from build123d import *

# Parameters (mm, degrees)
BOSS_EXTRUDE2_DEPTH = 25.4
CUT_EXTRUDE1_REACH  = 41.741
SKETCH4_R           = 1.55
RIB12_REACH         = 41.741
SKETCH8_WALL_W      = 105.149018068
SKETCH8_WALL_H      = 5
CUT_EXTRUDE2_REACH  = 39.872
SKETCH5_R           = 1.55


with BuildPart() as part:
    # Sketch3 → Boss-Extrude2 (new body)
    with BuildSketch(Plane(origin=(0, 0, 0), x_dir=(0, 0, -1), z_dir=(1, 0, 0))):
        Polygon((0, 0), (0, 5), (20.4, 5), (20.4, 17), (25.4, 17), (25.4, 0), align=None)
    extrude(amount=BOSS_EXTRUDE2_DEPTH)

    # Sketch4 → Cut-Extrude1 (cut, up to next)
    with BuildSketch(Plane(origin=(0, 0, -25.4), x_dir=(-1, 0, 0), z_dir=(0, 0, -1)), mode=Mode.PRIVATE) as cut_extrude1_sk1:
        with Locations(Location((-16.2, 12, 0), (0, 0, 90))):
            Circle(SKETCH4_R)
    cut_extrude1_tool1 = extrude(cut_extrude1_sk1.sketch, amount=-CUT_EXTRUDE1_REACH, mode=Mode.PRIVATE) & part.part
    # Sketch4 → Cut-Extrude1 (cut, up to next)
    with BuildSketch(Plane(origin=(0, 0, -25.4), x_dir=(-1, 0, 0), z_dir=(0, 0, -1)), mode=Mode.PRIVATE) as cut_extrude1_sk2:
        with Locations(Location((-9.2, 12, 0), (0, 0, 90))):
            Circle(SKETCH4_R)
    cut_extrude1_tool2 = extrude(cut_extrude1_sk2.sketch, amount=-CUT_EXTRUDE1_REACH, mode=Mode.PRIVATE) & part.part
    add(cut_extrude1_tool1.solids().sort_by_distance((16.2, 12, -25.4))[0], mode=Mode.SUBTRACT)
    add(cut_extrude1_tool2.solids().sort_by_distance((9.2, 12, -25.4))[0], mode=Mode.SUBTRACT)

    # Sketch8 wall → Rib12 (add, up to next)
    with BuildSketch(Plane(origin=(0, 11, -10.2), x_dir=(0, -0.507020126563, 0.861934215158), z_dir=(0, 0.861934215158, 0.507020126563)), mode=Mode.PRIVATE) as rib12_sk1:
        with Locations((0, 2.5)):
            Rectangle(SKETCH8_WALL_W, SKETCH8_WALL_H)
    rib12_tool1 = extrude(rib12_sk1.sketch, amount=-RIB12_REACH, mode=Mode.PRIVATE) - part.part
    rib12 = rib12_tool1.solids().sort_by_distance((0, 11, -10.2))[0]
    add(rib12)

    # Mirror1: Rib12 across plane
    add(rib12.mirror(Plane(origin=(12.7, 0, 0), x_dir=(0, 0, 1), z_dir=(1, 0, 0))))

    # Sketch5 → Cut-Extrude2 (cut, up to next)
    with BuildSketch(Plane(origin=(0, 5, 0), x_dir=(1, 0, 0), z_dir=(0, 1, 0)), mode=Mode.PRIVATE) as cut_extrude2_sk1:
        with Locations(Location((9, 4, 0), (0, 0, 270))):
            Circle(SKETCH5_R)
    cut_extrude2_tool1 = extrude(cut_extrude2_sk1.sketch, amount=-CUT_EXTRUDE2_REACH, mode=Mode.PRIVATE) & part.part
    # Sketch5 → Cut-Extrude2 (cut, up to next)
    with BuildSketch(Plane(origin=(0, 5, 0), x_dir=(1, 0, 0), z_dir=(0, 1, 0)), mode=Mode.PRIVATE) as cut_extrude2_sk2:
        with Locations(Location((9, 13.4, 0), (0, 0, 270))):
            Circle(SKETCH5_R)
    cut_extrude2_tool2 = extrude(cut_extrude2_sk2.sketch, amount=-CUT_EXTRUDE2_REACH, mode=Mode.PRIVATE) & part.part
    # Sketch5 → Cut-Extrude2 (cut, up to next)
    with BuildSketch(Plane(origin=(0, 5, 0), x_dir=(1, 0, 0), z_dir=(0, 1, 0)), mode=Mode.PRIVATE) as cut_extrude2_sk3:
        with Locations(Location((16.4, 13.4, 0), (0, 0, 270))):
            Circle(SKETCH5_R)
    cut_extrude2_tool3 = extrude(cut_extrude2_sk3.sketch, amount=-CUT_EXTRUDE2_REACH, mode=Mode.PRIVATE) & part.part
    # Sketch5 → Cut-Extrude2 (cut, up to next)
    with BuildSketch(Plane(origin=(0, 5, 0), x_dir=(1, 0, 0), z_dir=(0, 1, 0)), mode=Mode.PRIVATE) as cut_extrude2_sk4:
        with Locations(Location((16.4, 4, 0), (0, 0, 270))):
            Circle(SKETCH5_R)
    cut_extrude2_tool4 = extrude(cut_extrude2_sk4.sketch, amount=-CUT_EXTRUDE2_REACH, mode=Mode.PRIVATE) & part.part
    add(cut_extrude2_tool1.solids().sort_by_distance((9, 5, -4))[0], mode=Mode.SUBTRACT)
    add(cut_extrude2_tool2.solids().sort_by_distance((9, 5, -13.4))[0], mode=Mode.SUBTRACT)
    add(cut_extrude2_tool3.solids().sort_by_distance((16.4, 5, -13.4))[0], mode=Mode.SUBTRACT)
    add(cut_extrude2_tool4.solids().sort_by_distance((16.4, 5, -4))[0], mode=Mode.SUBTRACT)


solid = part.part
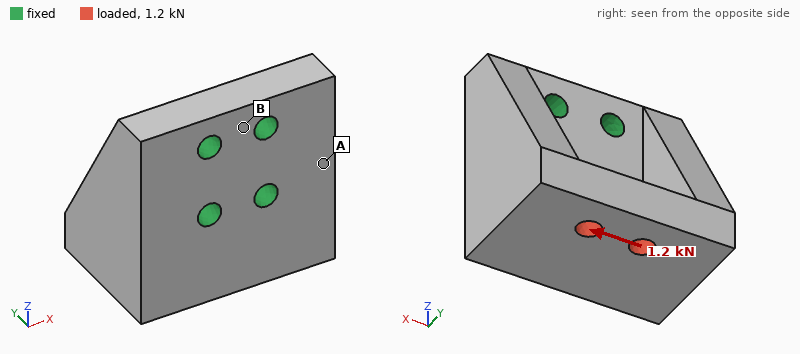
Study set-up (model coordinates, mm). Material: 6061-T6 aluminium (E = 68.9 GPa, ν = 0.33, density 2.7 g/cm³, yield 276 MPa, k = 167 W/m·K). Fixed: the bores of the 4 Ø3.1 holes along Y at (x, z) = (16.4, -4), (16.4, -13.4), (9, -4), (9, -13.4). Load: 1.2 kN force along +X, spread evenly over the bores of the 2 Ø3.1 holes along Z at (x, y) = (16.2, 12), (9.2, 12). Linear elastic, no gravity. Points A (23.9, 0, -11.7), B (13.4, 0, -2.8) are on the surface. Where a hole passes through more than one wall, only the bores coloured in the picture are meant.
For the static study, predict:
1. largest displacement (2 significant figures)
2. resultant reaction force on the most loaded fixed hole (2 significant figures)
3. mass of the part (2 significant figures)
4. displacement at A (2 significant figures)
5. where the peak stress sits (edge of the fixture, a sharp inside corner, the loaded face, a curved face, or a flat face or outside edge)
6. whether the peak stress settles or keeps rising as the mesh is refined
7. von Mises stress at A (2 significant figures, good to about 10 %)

35 µm
1.1 kN
16 g
8.0 µm
edge of the fixture
keeps rising
22 MPa
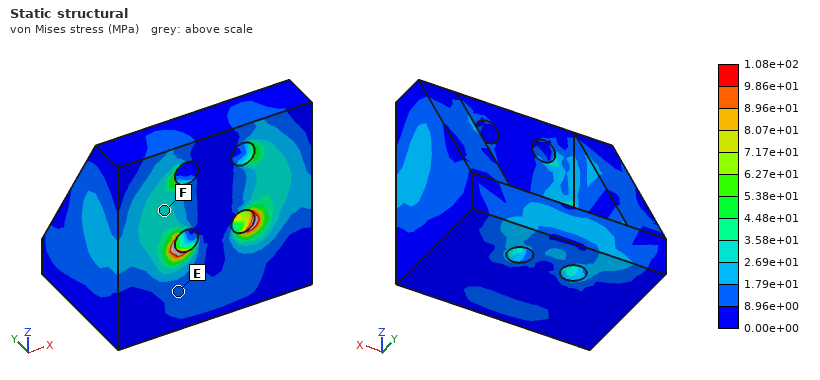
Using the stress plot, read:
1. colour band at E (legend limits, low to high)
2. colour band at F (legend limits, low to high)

8.96e+00 to 1.79e+01 MPa
2.69e+01 to 3.58e+01 MPa
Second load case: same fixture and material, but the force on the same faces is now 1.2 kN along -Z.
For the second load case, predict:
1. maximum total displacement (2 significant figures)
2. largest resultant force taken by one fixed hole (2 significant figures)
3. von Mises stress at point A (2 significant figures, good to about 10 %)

32 µm
600 N
16 MPa
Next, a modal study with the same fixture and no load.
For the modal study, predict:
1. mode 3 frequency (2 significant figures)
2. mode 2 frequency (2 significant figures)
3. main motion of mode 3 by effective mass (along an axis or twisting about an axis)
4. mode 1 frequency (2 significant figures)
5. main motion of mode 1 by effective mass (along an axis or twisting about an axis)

26 kHz
15 kHz
along X
13 kHz
along X
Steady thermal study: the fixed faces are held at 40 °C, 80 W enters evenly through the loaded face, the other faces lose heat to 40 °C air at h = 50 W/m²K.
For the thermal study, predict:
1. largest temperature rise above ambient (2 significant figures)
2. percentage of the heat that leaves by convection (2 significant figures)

59 K
3.4 %
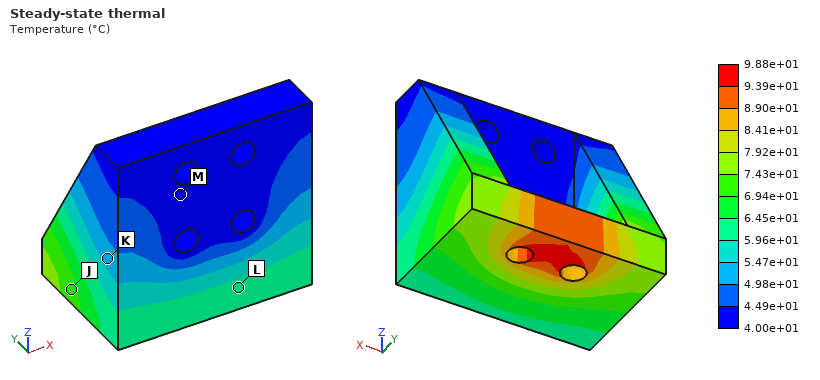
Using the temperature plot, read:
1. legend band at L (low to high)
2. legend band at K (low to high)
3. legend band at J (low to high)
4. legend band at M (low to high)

5.96e+01 to 6.45e+01 °C
4.98e+01 to 5.47e+01 °C
6.94e+01 to 7.43e+01 °C
4.00e+01 to 4.49e+01 °C
